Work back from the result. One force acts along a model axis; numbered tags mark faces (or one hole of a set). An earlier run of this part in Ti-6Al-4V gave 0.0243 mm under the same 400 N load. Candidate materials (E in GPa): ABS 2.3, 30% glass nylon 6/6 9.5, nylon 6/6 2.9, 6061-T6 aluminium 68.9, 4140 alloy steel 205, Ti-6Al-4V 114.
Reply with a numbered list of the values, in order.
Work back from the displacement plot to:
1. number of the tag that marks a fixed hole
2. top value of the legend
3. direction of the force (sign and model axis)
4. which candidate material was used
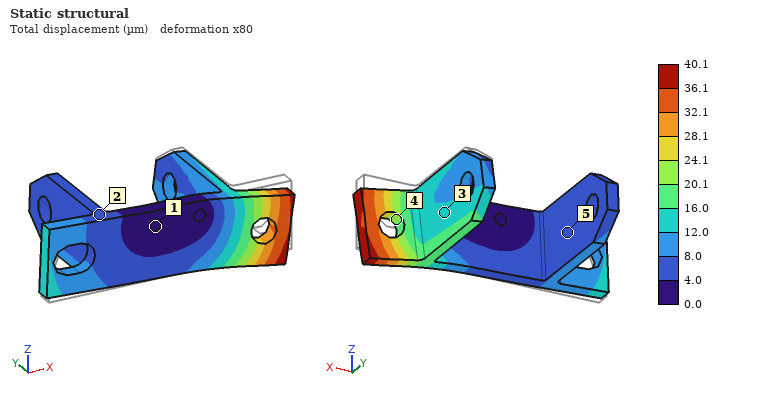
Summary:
1. 1
2. 40.1 µm
3. -Z
4. 6061-T6 aluminium
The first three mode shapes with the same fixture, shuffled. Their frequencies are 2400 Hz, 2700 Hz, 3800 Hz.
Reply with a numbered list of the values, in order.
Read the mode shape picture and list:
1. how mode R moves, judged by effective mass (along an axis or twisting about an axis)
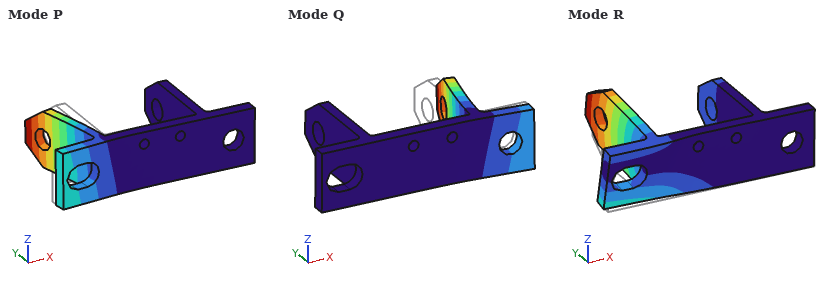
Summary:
1. along Z
